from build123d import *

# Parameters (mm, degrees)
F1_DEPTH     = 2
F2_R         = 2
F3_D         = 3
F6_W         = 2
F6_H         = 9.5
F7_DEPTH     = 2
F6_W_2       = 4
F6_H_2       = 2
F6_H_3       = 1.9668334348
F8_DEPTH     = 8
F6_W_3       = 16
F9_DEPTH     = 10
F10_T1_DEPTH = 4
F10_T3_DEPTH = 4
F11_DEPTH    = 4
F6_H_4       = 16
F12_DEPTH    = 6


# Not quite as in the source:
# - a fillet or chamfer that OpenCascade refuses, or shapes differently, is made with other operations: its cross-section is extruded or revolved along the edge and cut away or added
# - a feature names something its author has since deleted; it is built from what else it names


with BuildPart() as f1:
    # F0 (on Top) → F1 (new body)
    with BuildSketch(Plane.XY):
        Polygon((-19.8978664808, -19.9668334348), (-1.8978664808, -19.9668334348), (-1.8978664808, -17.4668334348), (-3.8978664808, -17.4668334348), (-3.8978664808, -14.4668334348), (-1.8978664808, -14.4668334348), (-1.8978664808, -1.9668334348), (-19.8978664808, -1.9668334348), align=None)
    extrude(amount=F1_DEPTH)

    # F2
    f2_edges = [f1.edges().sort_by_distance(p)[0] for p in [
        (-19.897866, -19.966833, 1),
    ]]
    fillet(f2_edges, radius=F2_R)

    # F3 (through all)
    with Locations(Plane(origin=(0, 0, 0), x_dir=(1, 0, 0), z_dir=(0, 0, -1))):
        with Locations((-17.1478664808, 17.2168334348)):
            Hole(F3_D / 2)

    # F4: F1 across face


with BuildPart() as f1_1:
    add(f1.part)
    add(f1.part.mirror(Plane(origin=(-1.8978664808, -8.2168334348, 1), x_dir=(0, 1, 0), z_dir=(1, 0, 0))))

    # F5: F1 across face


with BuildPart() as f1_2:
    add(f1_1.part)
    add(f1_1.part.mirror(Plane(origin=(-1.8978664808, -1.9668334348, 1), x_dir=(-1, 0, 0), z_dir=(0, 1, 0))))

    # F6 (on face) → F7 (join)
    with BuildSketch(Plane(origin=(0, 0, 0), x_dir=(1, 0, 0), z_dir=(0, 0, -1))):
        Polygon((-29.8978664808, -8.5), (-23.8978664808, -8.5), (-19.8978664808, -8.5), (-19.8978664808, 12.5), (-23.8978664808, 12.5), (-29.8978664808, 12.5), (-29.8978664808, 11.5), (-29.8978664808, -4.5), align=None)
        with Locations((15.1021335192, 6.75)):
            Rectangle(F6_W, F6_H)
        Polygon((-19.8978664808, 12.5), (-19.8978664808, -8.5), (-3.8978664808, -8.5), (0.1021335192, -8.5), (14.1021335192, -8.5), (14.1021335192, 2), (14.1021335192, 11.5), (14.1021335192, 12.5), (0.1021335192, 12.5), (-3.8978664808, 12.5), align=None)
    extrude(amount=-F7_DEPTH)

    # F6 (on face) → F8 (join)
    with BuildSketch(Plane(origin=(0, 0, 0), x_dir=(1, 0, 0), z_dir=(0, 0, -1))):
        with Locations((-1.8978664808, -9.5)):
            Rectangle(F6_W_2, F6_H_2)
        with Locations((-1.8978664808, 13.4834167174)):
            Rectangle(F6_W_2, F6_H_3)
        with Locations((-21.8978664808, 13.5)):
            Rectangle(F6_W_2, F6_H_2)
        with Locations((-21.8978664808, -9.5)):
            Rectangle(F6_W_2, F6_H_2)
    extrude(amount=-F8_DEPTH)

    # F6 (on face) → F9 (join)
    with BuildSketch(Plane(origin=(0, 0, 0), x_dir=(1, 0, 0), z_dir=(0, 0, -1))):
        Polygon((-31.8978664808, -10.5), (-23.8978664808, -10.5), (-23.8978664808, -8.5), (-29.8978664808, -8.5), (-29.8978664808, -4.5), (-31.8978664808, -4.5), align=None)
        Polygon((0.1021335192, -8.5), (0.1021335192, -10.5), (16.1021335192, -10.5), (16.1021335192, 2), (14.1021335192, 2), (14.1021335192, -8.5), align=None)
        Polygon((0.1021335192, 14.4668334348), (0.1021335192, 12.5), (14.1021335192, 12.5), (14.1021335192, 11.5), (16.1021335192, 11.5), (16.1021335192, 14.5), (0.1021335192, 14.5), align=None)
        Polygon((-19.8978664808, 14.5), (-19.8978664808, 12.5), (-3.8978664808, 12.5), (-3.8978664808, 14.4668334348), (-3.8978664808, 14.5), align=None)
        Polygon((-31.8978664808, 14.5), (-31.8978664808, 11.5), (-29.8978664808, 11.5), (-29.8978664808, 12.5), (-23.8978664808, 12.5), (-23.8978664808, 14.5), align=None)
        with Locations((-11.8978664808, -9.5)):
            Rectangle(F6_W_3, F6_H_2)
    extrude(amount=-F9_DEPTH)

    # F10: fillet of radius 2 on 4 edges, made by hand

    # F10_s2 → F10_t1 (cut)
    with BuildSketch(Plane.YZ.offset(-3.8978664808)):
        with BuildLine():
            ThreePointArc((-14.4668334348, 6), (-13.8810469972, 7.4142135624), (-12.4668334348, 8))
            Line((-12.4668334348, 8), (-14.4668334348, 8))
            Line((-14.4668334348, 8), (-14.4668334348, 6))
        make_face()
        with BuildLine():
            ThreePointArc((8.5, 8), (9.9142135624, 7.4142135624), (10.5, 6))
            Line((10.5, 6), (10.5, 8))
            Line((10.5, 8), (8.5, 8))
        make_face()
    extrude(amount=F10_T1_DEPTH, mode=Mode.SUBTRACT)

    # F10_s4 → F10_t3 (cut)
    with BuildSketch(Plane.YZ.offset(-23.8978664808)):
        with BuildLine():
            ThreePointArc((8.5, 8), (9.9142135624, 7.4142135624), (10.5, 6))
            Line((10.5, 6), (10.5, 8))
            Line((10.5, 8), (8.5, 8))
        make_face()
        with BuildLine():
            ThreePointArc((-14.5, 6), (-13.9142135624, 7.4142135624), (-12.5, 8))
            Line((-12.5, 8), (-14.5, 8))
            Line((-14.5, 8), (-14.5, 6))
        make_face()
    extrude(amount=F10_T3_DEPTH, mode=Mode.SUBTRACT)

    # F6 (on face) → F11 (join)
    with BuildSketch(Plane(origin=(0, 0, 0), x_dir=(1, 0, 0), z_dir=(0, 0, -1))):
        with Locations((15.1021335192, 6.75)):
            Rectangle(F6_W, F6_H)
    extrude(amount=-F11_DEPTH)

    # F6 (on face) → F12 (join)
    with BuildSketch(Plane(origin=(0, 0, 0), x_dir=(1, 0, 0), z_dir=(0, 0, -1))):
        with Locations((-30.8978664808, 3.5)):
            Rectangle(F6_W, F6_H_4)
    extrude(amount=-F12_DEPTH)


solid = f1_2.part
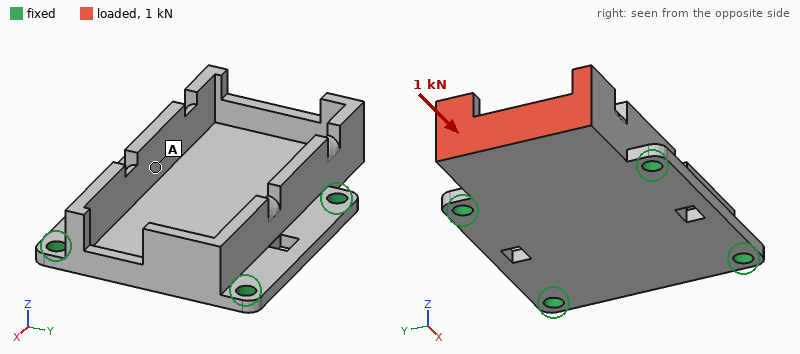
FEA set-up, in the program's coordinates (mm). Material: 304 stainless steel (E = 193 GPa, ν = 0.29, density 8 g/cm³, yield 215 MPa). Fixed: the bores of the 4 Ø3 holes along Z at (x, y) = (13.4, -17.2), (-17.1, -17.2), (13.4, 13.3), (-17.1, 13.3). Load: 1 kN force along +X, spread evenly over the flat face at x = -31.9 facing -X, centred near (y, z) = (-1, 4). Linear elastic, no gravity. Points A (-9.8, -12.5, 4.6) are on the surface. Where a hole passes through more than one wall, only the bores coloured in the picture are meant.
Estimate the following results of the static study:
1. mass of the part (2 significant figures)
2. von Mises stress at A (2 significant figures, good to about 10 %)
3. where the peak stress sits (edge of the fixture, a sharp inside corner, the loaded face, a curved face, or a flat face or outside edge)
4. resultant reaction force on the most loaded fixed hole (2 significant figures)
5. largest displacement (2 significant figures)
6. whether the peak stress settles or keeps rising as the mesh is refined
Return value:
40 g
9.8 MPa
edge of the fixture
320 N
16 µm
keeps rising
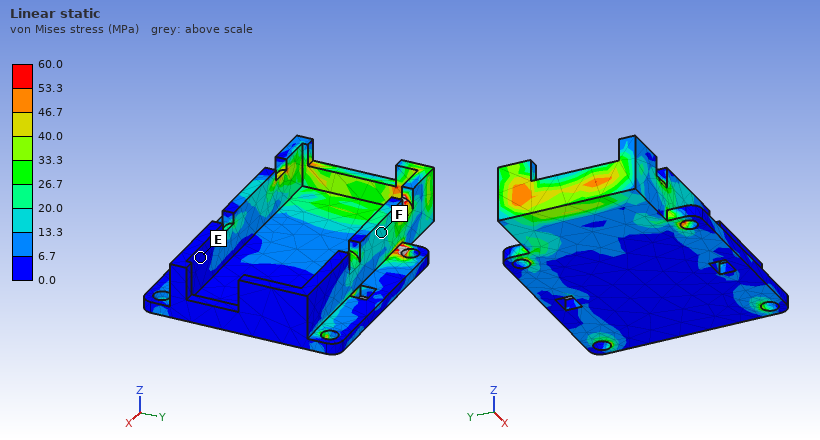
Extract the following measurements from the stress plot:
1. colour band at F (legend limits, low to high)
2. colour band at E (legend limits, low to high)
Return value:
13.3 to 20.0 MPa
0.0 to 6.7 MPa
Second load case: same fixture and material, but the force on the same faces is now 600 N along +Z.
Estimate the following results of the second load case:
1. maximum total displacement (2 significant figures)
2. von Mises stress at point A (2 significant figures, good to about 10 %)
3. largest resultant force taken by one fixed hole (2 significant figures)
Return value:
47 µm
22 MPa
480 N
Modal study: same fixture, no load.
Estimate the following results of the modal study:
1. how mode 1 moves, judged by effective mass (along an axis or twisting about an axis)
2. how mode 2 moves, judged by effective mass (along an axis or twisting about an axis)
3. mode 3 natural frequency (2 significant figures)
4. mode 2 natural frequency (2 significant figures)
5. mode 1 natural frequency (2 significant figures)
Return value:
along Z
along Z
13 kHz
9400 Hz
8200 Hz
